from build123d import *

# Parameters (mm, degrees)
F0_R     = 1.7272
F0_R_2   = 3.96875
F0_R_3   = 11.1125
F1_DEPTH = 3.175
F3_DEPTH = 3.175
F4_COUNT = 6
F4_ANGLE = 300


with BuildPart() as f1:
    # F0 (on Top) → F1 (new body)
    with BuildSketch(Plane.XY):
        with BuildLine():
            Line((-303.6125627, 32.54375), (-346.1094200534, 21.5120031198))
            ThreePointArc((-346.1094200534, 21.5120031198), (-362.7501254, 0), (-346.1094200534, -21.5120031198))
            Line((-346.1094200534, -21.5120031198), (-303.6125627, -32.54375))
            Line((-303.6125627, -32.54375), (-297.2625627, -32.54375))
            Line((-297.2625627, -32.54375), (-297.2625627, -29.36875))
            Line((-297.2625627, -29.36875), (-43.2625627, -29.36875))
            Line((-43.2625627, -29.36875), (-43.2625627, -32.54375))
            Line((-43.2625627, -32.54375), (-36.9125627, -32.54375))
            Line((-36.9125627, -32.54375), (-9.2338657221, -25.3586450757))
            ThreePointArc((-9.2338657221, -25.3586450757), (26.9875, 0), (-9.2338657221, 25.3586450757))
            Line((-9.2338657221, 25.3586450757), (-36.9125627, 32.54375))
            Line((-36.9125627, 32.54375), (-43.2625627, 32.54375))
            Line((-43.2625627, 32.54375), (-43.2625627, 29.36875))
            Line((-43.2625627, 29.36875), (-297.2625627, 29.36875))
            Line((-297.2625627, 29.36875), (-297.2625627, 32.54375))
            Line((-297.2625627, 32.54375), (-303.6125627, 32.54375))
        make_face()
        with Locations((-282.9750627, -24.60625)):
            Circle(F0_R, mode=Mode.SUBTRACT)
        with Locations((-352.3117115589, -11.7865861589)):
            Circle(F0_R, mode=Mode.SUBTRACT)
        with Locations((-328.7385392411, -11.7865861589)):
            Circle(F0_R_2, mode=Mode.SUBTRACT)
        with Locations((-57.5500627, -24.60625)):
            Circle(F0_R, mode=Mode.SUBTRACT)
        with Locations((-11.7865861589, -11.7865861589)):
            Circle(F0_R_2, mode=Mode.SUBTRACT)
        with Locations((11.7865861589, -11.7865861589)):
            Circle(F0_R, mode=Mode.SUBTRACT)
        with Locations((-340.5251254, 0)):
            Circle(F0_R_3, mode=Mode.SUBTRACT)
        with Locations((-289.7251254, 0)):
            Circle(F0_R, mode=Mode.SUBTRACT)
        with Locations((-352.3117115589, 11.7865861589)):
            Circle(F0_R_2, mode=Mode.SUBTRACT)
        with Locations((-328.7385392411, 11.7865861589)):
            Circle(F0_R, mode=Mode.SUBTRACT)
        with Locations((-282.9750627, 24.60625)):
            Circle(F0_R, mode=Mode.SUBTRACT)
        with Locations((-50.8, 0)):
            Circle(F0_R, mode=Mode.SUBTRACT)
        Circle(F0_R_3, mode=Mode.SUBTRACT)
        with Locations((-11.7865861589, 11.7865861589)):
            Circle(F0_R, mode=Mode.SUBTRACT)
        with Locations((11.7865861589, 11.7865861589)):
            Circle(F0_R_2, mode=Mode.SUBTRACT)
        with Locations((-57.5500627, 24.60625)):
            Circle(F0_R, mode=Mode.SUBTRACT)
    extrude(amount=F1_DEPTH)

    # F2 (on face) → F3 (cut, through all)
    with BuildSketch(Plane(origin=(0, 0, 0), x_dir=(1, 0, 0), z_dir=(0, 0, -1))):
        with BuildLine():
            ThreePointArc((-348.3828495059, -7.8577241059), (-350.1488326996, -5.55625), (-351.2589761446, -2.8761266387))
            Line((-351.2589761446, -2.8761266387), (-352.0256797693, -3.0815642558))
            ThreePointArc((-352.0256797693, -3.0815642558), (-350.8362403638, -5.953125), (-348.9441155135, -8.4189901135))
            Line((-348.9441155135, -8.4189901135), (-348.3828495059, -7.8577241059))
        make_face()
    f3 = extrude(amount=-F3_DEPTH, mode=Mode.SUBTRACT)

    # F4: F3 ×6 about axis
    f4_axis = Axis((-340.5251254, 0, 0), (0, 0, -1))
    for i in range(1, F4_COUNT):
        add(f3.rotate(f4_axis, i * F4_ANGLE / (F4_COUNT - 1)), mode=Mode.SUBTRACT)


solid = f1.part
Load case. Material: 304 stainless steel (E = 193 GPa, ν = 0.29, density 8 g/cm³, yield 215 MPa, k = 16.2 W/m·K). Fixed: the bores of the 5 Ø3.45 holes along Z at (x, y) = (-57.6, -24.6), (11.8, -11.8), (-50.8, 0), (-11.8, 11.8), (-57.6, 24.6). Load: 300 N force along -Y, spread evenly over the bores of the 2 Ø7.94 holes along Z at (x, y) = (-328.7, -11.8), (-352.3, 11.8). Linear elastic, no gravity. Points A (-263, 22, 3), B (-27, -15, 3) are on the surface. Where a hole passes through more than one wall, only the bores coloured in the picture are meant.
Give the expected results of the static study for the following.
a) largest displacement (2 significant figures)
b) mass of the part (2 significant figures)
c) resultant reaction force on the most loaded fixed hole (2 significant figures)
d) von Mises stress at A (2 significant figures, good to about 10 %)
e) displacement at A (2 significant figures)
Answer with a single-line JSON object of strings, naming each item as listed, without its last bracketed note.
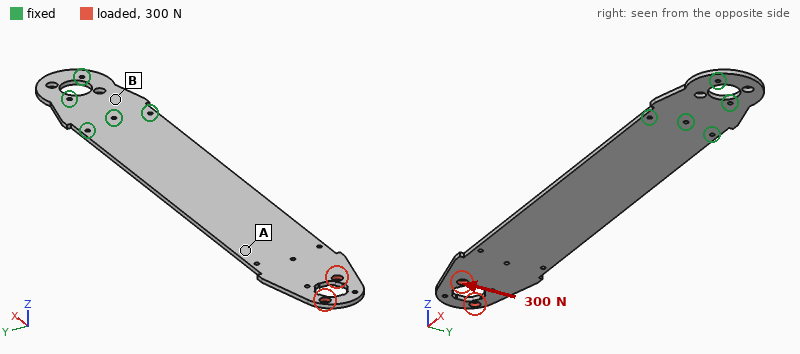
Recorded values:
{"largest displacement": "0.26 mm", "mass of the part": "530 g", "resultant reaction force on the most loaded fixed hole": "1.6 kN", "von Mises stress at A": "9.6 MPa", "displacement at A": "0.14 mm"}
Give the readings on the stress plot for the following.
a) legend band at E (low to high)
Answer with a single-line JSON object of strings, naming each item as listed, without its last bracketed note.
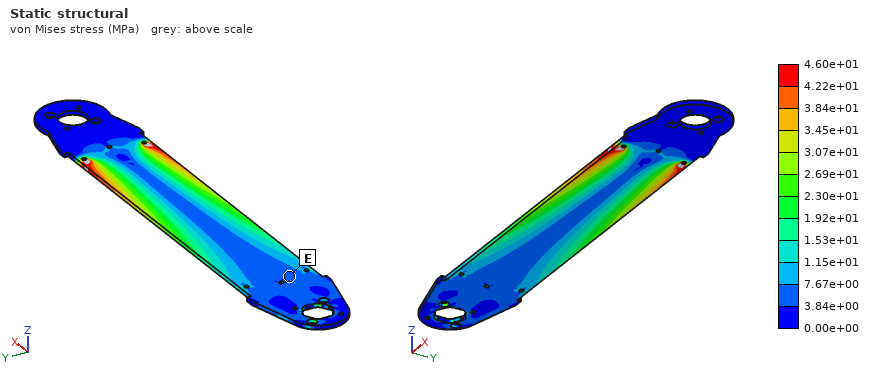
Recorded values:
{"legend band at E": "3.84e+00 to 7.67e+00 MPa"}
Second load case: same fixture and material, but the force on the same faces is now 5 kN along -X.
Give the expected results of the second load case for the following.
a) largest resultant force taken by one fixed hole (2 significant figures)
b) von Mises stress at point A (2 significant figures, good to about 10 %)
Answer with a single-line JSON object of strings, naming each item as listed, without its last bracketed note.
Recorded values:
{"largest resultant force taken by one fixed hole": "1.6 kN", "von Mises stress at point A": "27 MPa"}
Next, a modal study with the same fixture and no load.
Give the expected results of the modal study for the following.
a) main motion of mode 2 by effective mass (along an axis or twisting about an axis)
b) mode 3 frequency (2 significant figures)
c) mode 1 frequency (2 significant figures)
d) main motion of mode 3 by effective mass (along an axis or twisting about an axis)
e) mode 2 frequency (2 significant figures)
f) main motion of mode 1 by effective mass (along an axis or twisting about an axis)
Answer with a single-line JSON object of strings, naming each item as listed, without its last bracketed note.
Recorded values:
{"main motion of mode 2 by effective mass": "along Z", "mode 3 frequency": "300 Hz", "mode 1 frequency": "30 Hz", "main motion of mode 3 by effective mass": "twisting about X", "mode 2 frequency": "190 Hz", "main motion of mode 1 by effective mass": "along Z"}
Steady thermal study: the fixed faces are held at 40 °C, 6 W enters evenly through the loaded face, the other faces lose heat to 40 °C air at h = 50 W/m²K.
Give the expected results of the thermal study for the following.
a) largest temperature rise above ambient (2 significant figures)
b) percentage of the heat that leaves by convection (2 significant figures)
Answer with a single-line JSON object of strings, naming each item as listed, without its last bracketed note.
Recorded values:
{"largest temperature rise above ambient": "59 K", "percentage of the heat that leaves by convection": "100 %"}
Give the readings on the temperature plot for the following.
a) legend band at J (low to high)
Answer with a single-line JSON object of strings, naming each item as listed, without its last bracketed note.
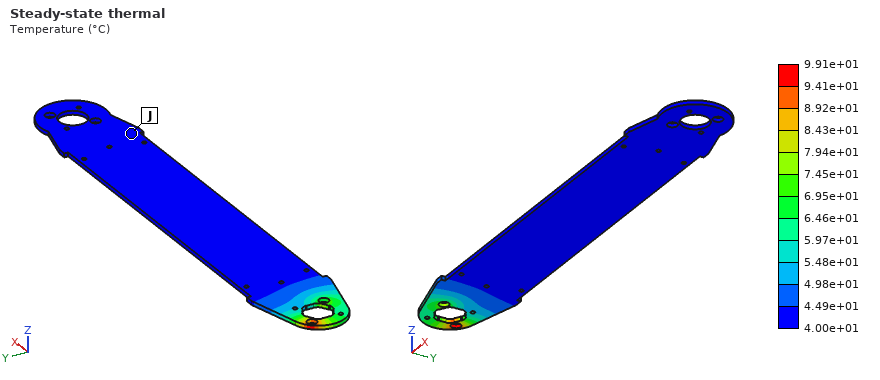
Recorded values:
{"legend band at J": "4.00e+01 to 4.49e+01 °C"}
